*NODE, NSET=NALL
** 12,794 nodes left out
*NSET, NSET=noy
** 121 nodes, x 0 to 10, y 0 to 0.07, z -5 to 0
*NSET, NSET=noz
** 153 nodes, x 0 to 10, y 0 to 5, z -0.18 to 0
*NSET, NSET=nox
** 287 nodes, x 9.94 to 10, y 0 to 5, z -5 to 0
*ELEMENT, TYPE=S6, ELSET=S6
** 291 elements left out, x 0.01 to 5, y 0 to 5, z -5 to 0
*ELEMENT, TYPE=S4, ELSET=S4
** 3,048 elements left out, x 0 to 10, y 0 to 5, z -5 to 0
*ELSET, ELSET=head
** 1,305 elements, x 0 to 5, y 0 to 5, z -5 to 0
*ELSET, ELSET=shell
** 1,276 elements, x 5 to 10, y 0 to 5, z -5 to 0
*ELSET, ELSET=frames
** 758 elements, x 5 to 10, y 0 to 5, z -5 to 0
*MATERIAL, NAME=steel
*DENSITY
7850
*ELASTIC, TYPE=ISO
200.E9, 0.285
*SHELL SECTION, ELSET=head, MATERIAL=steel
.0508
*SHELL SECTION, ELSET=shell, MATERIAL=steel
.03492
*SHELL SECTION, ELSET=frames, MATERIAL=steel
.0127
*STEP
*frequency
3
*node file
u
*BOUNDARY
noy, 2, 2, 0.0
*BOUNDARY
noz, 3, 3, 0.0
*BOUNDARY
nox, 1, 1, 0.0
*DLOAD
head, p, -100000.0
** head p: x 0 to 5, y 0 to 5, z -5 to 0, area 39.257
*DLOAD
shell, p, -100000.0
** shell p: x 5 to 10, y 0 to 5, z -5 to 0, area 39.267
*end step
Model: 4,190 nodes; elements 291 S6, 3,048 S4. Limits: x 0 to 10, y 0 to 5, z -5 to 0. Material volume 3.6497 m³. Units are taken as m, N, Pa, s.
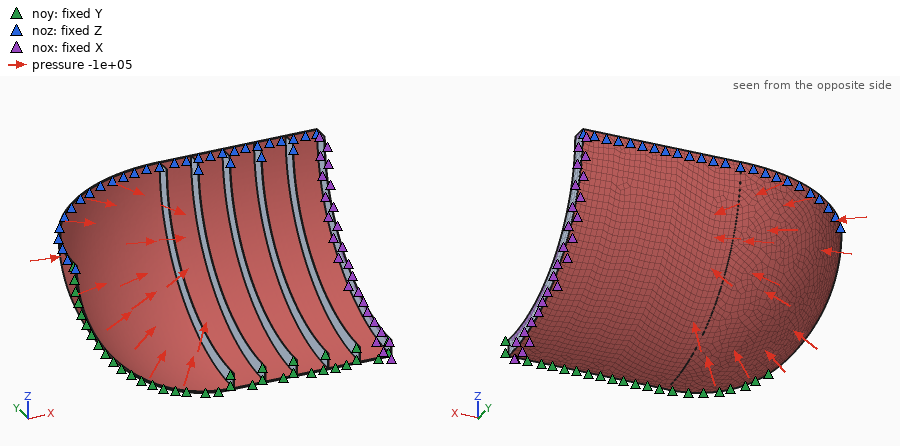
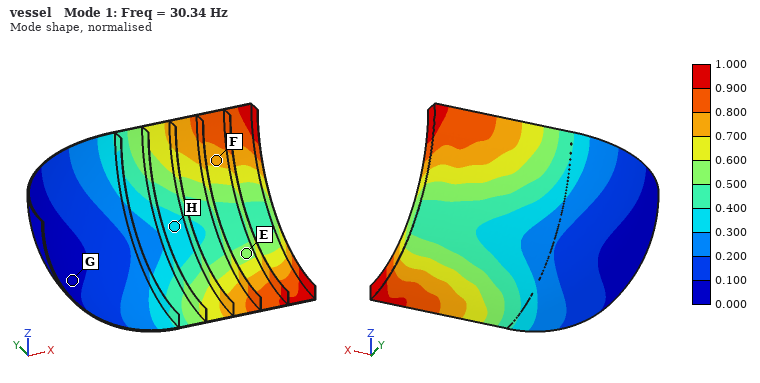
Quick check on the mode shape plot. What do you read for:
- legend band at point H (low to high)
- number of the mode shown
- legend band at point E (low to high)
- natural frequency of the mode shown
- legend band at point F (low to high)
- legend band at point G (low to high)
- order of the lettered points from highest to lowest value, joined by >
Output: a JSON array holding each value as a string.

["0.300 to 0.400", "1", "0.500 to 0.600", "30.34 Hz", "0.700 to 0.800", "0.000 to 0.100", "F > E > H > G"]
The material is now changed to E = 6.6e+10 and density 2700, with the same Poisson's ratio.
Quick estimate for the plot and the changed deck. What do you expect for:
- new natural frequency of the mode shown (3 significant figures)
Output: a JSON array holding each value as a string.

["29.7 Hz"]
